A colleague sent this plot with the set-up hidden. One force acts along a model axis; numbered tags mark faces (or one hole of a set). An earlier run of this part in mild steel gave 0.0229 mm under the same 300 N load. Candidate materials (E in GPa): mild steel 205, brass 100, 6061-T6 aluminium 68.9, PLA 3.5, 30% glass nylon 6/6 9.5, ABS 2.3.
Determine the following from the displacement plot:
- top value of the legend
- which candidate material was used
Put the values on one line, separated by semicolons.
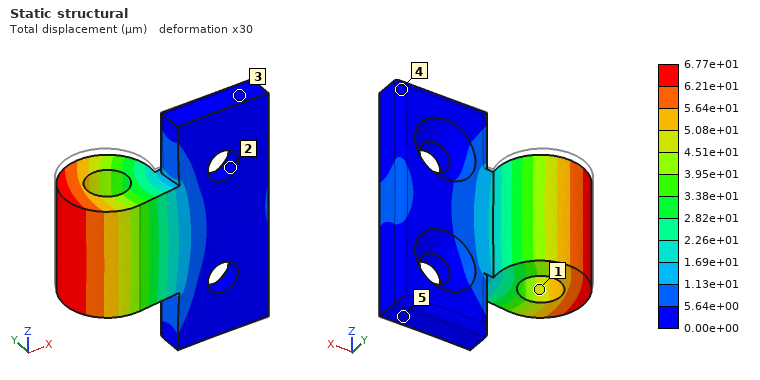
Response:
6.77e+01 µm; 6061-T6 aluminium
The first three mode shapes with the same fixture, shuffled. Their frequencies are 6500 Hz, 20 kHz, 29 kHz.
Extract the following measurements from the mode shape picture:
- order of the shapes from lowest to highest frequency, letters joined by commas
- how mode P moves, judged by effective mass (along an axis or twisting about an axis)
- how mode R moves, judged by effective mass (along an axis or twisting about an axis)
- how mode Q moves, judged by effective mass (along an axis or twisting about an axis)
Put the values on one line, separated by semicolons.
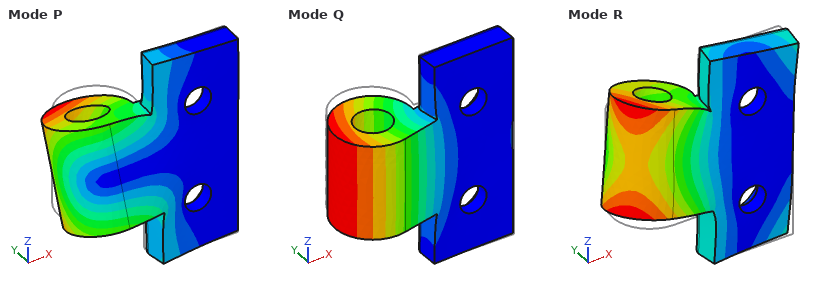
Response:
Q, P, R; along Z; along Z; along Y
